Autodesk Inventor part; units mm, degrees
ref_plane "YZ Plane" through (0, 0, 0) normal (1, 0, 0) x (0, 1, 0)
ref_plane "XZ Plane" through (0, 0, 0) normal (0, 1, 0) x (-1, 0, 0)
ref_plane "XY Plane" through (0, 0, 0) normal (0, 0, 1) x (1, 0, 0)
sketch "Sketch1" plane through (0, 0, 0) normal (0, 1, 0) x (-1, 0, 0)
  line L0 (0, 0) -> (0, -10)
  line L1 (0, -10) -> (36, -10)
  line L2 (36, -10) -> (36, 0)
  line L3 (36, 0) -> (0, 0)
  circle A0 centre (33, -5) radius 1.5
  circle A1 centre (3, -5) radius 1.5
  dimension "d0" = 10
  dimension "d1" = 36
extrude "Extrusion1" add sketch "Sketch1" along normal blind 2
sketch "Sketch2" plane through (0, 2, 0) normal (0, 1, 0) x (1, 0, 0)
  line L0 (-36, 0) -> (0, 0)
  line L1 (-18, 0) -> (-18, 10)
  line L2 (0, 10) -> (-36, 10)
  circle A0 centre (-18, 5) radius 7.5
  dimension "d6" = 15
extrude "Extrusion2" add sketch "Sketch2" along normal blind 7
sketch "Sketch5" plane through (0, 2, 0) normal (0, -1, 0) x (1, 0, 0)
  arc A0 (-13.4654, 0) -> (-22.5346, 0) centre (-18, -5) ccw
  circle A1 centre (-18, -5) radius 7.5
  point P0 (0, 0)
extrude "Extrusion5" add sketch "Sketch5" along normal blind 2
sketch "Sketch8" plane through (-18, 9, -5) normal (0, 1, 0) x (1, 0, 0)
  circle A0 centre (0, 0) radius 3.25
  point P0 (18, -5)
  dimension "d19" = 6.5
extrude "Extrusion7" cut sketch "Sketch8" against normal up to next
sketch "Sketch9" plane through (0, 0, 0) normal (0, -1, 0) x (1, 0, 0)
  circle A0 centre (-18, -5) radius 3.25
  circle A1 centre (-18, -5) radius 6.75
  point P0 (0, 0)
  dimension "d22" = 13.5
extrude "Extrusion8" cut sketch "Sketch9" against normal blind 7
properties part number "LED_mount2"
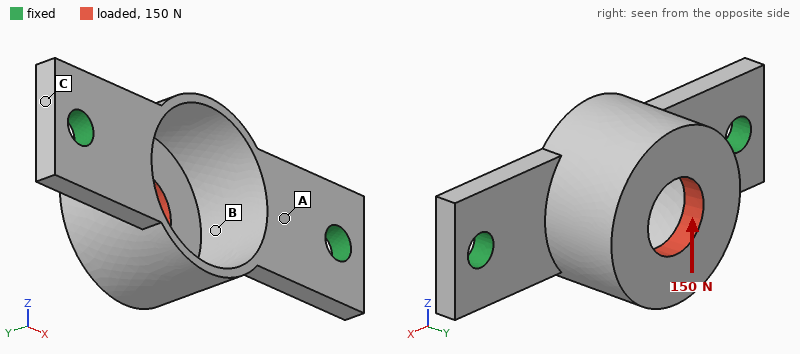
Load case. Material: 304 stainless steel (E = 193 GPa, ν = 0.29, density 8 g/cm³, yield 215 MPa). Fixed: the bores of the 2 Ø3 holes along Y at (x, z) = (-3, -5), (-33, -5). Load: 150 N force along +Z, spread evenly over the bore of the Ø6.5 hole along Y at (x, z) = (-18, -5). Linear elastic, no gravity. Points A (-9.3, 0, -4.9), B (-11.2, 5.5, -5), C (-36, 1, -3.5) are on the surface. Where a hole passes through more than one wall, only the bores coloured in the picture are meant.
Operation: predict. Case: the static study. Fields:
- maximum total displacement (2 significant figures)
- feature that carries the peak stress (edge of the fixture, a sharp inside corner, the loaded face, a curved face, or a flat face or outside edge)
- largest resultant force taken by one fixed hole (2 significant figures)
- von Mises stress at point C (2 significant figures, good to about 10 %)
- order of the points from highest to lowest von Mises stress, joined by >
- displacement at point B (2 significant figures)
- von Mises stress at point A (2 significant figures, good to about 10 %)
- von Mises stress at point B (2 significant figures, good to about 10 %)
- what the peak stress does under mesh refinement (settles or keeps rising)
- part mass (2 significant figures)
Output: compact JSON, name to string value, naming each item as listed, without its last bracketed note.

{"maximum total displacement": "29 µm", "feature that carries the peak stress": "edge of the fixture", "largest resultant force taken by one fixed hole": "75 N", "von Mises stress at point C": "20 MPa", "order of the points from highest to lowest von Mises stress, joined by >": "A > B > C", "displacement at point B": "13 µm", "von Mises stress at point A": "74 MPa", "von Mises stress at point B": "42 MPa", "what the peak stress does under mesh refinement": "keeps rising", "part mass": "7.5 g"}
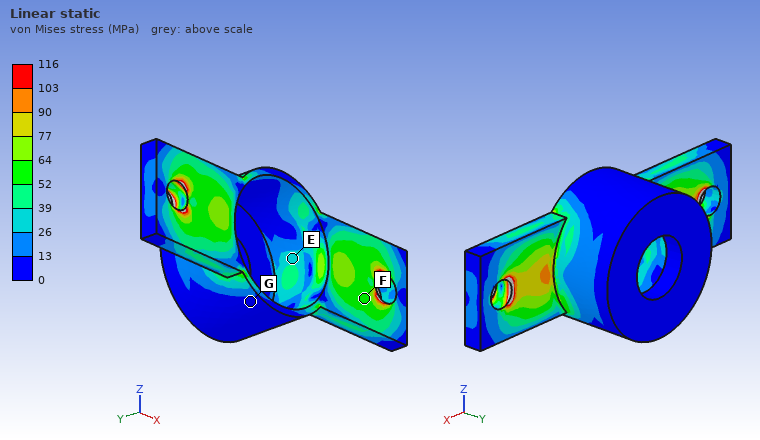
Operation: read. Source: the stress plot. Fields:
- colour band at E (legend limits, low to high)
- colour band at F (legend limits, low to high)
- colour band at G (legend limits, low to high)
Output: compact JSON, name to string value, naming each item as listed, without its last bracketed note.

{"colour band at E": "26 to 39 MPa", "colour band at F": "52 to 64 MPa", "colour band at G": "0 to 13 MPa"}
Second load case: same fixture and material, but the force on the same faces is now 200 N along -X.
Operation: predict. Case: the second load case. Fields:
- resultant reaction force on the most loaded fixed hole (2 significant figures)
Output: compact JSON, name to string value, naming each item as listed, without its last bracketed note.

{"resultant reaction force on the most loaded fixed hole": "120 N"}
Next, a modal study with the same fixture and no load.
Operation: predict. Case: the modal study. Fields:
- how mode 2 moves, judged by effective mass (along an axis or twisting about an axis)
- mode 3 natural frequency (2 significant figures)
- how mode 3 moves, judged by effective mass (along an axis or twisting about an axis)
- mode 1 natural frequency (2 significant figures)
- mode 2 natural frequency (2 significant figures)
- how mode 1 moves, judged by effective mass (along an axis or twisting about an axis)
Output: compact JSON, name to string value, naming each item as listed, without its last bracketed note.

{"how mode 2 moves, judged by effective mass": "along Y", "mode 3 natural frequency": "15 kHz", "how mode 3 moves, judged by effective mass": "along X", "mode 1 natural frequency": "6800 Hz", "mode 2 natural frequency": "12 kHz", "how mode 1 moves, judged by effective mass": "along Z"}
